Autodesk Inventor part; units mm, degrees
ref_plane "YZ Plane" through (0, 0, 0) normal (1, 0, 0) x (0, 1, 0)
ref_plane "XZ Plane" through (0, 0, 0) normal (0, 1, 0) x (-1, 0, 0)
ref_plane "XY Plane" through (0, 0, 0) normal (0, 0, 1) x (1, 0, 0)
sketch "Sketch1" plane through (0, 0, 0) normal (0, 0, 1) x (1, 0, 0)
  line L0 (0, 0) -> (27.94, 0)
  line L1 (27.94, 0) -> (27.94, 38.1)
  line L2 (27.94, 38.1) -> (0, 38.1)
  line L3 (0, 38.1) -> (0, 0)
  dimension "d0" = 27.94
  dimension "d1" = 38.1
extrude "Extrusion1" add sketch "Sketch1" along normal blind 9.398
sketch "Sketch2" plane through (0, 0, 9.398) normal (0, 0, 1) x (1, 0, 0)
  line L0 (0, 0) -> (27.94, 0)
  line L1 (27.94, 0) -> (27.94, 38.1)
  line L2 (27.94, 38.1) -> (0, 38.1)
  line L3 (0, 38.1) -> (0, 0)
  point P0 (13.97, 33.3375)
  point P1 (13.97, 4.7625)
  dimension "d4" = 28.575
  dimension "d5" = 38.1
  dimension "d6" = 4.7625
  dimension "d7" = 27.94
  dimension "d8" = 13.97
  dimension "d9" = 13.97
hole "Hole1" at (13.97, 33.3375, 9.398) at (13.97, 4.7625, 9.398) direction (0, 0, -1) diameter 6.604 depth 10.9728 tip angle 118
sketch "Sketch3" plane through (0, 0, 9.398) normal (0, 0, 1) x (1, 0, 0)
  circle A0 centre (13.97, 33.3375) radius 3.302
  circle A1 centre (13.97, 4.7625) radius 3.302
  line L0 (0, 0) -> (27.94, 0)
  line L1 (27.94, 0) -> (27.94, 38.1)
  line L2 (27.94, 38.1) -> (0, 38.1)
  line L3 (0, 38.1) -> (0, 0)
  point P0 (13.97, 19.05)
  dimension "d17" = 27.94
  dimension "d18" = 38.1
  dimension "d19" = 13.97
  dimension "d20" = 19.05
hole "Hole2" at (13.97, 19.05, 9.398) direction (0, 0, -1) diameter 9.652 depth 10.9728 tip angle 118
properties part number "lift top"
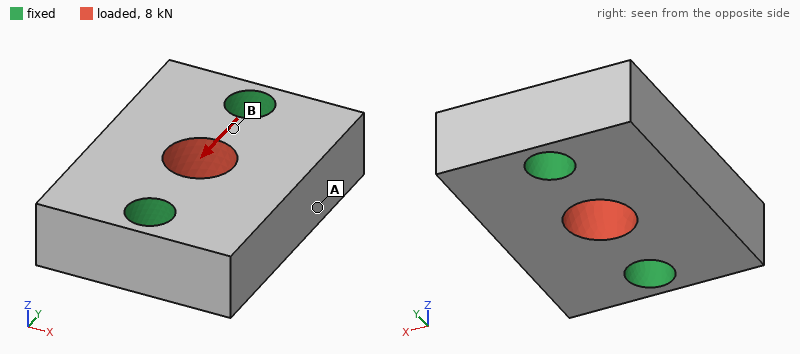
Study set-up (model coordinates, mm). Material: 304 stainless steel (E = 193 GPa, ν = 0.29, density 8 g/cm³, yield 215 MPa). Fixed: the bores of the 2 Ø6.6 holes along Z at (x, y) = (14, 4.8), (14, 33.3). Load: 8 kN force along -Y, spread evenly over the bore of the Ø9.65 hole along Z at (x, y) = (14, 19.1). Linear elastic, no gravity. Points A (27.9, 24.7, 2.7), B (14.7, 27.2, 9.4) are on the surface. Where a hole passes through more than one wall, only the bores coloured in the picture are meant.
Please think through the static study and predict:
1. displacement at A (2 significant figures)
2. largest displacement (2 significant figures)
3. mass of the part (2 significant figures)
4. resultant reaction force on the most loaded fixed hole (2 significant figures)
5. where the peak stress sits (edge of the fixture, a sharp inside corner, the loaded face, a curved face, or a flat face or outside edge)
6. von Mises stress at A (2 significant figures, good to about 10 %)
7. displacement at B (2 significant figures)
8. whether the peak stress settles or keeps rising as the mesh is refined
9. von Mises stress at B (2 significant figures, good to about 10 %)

1.00 µm
2.0 µm
69 g
4.0 kN
edge of the fixture
7.9 MPa
0.66 µm
keeps rising
38 MPa
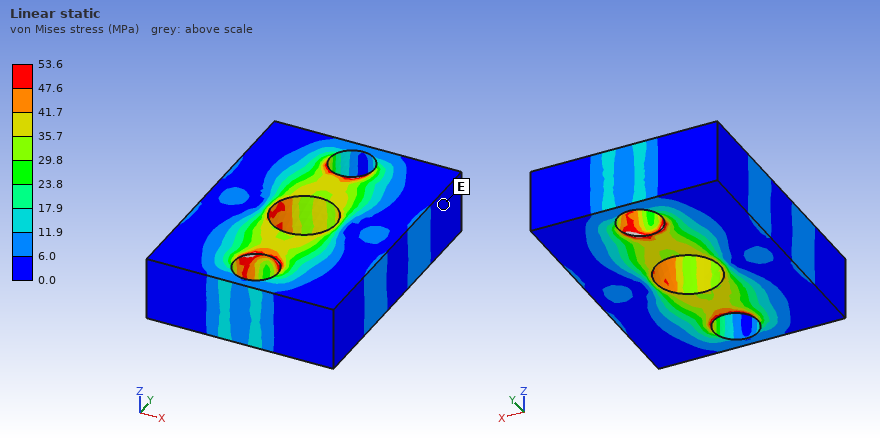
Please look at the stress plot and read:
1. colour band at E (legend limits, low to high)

0.0 to 6.0 MPa
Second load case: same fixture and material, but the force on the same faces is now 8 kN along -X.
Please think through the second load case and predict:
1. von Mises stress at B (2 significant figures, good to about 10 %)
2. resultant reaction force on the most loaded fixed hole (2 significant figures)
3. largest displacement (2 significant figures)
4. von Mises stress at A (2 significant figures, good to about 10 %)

41 MPa
4.0 kN
3.5 µm
23 MPa
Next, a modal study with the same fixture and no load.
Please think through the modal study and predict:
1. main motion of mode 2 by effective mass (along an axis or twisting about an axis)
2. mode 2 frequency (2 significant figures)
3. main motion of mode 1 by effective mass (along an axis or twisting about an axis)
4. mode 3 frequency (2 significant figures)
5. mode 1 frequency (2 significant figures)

along Z
30 kHz
twisting about Y
42 kHz
27 kHz
